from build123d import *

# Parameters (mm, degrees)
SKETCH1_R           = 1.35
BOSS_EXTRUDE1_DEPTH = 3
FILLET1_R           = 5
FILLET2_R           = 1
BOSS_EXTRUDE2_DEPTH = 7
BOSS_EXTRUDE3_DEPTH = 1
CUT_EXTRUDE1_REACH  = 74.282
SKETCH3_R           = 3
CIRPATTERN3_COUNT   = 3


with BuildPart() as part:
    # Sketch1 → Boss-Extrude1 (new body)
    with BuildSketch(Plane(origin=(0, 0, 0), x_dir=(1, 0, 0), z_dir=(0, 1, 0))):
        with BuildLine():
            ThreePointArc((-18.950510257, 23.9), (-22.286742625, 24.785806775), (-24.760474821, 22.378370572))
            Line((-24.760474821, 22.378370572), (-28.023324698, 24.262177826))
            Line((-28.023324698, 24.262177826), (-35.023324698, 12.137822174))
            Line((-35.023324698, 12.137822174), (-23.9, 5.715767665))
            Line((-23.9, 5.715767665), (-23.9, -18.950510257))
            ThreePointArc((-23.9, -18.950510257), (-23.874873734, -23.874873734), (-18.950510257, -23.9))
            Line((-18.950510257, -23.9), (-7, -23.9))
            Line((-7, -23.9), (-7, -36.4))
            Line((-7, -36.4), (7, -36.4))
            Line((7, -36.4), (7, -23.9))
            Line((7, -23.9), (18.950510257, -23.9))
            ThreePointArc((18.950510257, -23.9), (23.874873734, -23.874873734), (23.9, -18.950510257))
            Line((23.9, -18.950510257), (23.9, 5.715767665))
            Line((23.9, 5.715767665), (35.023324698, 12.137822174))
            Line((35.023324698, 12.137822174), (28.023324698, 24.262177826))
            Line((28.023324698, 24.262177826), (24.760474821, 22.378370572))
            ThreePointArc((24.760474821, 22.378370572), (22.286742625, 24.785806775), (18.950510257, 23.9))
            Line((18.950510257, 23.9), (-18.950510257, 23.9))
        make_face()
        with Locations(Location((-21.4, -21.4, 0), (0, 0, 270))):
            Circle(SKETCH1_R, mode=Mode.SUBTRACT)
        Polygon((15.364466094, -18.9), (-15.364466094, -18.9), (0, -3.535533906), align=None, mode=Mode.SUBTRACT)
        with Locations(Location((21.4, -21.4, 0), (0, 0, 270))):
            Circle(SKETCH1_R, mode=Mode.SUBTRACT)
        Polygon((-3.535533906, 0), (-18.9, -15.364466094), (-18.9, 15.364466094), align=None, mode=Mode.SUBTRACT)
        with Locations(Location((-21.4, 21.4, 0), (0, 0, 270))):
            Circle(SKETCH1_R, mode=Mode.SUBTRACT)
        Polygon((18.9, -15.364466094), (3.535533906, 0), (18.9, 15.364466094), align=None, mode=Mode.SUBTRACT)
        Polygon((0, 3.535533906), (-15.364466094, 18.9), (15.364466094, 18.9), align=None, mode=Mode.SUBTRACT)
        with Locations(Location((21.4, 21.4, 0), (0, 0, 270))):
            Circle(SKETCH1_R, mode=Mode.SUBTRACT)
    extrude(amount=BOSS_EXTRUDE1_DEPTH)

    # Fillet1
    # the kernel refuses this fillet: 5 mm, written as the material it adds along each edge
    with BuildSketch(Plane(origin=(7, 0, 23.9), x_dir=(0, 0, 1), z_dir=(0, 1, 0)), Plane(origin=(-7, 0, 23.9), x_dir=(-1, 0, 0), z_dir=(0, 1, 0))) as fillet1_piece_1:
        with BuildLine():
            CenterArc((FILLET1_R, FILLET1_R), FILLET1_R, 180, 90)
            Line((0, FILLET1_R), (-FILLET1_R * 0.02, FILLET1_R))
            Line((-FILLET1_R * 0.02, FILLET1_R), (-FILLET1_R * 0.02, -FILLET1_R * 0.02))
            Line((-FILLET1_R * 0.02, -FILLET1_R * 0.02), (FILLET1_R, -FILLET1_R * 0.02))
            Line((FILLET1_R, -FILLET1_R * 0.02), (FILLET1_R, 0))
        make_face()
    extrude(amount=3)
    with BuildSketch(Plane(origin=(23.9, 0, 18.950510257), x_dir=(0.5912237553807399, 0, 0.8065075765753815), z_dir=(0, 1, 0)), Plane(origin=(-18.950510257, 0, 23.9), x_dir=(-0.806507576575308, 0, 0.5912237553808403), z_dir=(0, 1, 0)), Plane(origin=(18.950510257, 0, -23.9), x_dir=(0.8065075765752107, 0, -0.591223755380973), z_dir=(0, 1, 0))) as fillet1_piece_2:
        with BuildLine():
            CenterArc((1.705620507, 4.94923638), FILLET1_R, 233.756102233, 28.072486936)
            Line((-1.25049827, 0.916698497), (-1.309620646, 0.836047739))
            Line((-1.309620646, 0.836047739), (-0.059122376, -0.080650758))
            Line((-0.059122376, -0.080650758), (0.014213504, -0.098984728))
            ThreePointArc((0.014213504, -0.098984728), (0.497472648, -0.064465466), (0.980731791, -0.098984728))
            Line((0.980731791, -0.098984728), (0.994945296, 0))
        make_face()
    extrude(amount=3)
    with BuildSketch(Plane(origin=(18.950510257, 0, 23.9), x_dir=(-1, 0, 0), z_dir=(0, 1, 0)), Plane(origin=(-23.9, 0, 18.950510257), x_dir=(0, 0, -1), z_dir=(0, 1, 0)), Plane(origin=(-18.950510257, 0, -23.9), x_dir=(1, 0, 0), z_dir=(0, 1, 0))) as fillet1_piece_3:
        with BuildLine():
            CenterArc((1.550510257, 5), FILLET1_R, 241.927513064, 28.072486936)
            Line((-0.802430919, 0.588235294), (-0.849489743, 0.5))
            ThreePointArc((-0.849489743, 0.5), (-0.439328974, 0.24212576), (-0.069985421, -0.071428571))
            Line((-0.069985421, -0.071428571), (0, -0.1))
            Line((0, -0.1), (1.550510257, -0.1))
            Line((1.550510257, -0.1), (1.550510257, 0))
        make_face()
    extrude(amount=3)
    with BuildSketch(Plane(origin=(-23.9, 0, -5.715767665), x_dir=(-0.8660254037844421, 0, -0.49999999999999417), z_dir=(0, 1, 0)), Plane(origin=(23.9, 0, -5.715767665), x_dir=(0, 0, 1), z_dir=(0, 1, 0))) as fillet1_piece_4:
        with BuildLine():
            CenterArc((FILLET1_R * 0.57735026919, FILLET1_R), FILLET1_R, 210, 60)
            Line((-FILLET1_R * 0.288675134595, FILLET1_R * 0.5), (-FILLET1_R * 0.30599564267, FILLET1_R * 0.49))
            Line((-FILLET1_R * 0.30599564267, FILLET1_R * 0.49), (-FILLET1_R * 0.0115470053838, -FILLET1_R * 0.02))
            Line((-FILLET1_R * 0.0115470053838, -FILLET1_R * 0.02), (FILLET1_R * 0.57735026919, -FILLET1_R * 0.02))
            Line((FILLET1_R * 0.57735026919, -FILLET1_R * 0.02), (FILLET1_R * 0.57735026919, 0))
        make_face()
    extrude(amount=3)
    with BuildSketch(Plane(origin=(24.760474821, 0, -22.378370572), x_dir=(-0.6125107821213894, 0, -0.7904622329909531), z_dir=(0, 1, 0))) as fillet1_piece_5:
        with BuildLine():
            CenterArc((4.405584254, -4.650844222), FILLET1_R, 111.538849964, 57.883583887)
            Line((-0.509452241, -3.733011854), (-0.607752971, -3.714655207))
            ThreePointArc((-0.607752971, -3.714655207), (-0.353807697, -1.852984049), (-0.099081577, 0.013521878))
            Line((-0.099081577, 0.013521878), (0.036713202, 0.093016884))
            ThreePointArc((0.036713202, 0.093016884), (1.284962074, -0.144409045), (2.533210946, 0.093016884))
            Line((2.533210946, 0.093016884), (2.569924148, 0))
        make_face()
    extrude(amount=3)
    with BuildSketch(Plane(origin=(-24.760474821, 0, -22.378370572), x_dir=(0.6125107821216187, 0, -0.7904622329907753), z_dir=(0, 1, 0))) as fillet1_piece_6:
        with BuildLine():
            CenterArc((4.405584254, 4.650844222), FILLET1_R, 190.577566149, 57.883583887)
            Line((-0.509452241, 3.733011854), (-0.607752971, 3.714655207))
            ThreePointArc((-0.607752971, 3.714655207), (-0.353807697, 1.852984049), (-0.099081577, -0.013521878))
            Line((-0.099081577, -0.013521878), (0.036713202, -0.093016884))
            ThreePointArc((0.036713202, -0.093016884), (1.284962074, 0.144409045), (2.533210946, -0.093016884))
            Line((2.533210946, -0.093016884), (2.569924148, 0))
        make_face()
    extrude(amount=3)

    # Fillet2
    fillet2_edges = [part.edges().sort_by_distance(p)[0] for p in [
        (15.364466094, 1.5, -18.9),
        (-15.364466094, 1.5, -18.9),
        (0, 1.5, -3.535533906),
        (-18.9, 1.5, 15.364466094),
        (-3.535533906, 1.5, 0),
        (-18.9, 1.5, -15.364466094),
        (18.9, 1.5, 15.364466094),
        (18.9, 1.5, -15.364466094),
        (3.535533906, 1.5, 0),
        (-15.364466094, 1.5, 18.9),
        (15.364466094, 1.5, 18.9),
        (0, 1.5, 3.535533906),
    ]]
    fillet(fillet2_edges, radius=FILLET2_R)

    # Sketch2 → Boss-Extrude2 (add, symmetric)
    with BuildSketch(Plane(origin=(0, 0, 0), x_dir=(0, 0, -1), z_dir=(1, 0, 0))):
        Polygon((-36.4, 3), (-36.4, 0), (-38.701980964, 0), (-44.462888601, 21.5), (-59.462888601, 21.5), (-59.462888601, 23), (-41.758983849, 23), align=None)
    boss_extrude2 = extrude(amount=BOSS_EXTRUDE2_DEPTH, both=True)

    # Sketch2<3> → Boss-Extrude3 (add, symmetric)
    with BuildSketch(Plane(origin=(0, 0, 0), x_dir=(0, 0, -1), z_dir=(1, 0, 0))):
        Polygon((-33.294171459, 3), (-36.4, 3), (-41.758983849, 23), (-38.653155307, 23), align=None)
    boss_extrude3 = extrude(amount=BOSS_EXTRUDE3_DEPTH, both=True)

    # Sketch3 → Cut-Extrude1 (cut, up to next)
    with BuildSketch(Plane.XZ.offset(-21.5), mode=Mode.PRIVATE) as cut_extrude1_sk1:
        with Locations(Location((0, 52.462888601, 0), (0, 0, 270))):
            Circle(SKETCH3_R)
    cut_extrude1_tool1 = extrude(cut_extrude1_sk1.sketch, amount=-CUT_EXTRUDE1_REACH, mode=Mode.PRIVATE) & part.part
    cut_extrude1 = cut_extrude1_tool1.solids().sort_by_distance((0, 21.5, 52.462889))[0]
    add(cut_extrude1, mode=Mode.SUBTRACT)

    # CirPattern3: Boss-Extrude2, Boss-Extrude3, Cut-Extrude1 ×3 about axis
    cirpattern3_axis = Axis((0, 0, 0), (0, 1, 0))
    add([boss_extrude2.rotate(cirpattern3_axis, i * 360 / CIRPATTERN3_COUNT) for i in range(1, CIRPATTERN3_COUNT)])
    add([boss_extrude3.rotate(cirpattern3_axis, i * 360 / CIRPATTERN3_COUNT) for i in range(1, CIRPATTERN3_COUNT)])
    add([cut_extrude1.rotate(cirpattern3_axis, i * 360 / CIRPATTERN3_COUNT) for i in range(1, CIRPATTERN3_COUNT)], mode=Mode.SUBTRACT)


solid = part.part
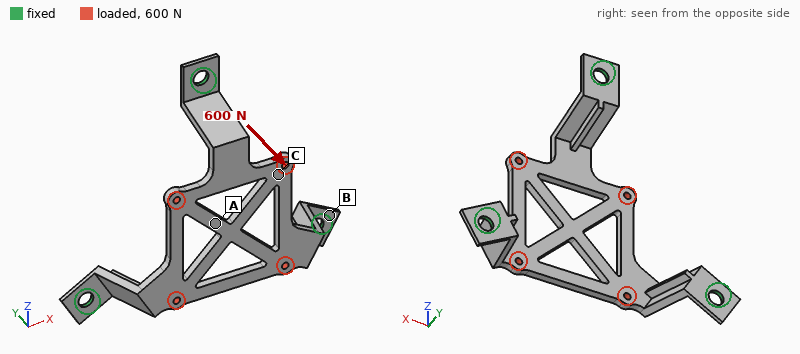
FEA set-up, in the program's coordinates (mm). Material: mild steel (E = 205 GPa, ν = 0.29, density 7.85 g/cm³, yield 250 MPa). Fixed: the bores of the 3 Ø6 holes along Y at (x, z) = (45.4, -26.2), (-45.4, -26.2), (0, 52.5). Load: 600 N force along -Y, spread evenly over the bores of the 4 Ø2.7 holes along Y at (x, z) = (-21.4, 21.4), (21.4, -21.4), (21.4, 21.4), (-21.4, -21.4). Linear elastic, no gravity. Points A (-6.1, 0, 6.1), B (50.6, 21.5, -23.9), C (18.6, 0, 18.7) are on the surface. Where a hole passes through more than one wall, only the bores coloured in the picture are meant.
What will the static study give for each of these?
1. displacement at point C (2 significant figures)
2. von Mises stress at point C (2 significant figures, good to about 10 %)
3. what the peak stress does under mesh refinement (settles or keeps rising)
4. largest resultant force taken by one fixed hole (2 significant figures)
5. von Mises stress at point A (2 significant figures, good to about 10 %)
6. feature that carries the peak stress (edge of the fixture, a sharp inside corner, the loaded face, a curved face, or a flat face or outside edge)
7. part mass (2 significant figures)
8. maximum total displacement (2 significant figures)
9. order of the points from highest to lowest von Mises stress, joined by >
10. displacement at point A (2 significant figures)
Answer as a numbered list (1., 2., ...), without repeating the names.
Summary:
1. 0.080 mm
2. 81 MPa
3. keeps rising
4. 280 N
5. 39 MPa
6. edge of the fixture
7. 75 g
8. 0.11 mm
9. C > A > B
10. 0.043 mm
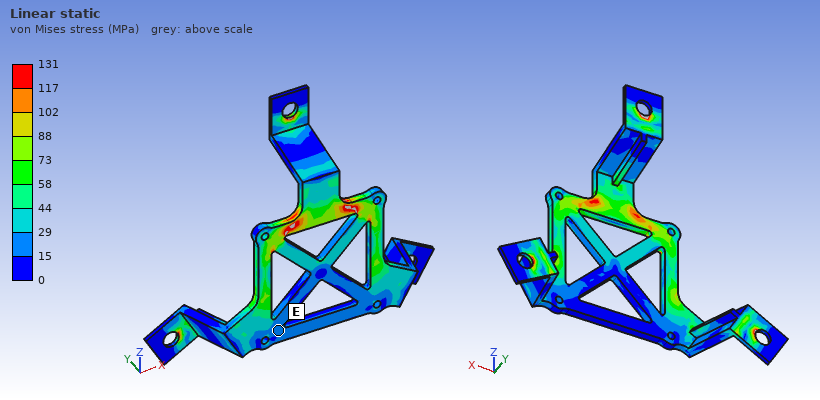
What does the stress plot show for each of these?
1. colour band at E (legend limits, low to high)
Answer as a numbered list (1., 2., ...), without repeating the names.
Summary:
1. 15 to 29 MPa
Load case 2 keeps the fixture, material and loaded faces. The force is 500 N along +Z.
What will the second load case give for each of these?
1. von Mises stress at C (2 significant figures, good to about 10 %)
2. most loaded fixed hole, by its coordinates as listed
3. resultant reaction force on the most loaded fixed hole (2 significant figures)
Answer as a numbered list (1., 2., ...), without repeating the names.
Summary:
1. 24 MPa
2. (0, 52.5)
3. 230 N
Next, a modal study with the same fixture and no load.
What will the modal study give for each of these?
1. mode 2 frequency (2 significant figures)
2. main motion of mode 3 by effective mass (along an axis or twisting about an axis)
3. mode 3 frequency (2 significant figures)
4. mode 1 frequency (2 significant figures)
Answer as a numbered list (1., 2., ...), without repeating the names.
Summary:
1. 1700 Hz
2. twisting about Y
3. 2400 Hz
4. 1700 Hz
